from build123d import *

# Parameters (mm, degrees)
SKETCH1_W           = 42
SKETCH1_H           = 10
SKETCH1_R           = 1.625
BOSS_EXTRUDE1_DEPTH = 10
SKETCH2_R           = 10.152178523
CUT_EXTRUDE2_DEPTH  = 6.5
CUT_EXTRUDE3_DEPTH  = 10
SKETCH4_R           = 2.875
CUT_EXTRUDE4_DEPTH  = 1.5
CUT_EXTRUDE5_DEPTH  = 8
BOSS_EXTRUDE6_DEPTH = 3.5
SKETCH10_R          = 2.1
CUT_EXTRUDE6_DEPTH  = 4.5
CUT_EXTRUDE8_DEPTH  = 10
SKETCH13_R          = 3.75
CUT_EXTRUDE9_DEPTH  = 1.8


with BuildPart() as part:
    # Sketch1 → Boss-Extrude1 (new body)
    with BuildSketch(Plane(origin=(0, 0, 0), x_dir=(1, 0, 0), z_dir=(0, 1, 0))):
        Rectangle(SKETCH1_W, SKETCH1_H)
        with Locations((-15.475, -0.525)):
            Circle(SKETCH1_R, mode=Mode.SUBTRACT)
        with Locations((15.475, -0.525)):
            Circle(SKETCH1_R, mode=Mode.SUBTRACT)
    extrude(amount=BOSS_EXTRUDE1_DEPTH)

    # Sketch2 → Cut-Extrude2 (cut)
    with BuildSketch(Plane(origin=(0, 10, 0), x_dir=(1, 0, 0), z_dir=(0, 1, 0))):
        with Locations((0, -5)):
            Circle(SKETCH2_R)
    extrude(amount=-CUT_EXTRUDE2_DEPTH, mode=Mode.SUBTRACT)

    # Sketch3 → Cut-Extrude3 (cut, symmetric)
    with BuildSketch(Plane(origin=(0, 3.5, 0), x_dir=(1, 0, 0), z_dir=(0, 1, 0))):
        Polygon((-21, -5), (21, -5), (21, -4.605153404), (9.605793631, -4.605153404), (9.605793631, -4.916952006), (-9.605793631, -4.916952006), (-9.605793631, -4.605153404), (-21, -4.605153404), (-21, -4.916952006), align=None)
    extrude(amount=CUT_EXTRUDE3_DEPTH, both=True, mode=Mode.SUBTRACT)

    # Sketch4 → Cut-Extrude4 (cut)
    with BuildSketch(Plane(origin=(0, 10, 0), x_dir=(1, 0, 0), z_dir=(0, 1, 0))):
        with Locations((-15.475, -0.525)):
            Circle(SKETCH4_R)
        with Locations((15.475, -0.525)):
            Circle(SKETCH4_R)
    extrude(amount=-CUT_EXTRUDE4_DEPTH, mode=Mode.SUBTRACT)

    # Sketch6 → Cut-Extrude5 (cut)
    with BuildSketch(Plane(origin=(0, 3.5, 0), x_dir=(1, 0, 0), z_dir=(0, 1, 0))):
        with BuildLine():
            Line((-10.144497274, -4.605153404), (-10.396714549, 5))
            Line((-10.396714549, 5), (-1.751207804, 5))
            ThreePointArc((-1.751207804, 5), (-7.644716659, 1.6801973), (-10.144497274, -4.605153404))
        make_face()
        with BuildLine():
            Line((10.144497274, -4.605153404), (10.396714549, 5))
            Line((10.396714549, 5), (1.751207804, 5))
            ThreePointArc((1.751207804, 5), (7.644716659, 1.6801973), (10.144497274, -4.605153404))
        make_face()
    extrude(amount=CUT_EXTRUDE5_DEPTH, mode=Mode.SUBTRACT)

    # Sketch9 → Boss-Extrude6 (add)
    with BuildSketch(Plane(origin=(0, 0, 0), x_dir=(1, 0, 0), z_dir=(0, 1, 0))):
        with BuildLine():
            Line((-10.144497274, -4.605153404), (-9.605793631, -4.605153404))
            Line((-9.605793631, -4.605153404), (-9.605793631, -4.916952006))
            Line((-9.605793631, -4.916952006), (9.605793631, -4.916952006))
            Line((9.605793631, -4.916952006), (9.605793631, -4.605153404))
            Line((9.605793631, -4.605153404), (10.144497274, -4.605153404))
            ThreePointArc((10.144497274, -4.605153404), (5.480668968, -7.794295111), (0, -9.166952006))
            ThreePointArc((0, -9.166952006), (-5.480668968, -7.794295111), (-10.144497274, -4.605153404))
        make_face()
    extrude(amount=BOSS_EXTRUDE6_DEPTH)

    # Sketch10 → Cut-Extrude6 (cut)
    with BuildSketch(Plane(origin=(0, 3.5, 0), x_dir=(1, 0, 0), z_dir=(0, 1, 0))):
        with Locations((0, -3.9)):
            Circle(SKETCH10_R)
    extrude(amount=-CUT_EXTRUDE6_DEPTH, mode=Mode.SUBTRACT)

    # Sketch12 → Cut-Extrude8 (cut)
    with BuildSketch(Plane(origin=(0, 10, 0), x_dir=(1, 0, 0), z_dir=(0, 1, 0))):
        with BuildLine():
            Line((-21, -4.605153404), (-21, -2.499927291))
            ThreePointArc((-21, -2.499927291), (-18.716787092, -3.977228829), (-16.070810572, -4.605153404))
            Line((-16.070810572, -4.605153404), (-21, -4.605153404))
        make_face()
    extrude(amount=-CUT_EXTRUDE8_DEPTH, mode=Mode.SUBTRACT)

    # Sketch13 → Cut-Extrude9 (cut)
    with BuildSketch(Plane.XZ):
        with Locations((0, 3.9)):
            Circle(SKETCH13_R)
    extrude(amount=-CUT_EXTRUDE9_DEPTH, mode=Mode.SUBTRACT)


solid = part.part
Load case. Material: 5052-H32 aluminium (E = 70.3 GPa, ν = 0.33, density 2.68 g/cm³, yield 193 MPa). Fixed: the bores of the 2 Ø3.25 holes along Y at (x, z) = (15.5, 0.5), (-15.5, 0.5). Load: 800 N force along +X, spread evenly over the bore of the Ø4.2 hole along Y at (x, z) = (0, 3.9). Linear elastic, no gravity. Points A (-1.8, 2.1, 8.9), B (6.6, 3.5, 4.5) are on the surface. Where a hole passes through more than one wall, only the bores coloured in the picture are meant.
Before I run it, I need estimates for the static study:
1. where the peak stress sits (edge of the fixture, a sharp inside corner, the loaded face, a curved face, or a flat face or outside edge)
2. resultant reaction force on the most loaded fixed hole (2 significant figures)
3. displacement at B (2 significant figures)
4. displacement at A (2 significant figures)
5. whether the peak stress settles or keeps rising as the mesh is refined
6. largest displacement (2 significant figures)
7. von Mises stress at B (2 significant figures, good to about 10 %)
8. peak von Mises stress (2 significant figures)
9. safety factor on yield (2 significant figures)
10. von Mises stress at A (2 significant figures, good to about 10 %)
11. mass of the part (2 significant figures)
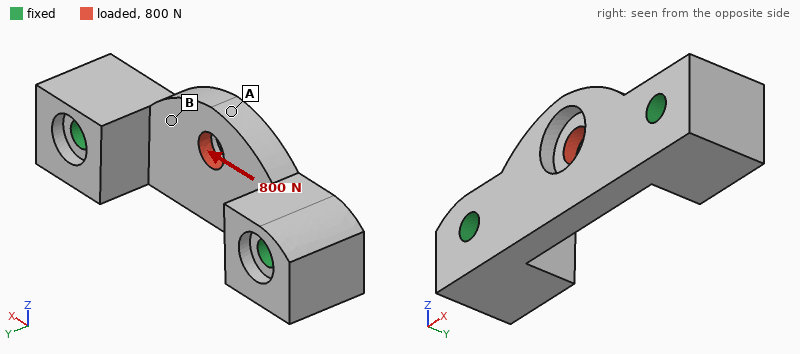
the loaded face
410 N
2.7 µm
3.4 µm
settles
5.5 µm
30 MPa
68 MPa
2.8
10 MPa
7.0 g
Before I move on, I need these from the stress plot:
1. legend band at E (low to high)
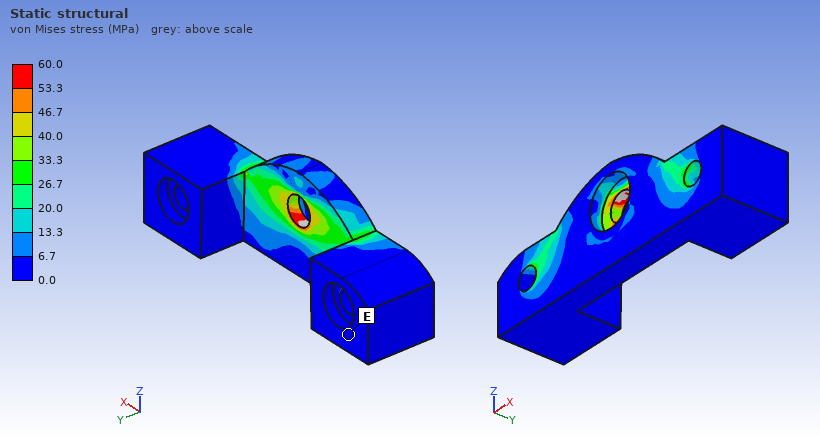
0.0 to 6.7 MPa
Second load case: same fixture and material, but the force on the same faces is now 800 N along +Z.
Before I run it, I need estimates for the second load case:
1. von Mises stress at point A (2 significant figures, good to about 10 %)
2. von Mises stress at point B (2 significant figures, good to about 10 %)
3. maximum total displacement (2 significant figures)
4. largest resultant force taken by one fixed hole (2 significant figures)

42 MPa
32 MPa
15 µm
400 N
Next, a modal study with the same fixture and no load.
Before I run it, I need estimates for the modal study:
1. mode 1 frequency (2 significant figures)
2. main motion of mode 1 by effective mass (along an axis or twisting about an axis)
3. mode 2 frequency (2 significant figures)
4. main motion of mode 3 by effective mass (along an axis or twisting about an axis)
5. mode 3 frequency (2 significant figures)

24 kHz
along Y
33 kHz
along Z
37 kHz
